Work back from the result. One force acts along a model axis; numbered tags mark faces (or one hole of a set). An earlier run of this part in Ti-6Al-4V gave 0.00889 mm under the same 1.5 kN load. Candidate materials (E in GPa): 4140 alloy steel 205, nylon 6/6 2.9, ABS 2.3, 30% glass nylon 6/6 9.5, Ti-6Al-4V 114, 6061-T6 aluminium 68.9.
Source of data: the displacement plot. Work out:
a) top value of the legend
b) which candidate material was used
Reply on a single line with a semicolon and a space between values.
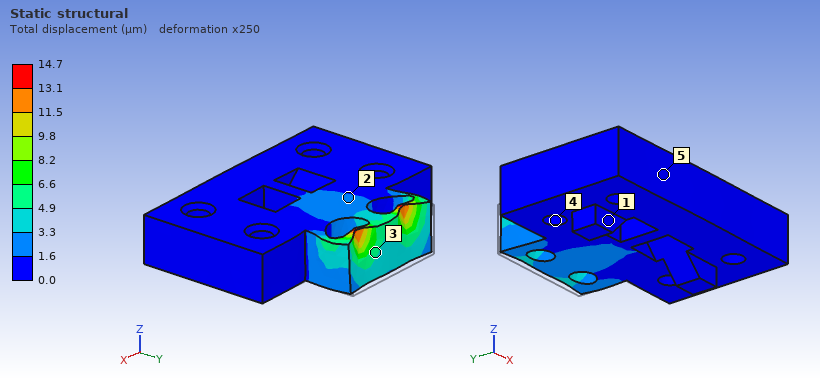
14.7 µm; 6061-T6 aluminium
